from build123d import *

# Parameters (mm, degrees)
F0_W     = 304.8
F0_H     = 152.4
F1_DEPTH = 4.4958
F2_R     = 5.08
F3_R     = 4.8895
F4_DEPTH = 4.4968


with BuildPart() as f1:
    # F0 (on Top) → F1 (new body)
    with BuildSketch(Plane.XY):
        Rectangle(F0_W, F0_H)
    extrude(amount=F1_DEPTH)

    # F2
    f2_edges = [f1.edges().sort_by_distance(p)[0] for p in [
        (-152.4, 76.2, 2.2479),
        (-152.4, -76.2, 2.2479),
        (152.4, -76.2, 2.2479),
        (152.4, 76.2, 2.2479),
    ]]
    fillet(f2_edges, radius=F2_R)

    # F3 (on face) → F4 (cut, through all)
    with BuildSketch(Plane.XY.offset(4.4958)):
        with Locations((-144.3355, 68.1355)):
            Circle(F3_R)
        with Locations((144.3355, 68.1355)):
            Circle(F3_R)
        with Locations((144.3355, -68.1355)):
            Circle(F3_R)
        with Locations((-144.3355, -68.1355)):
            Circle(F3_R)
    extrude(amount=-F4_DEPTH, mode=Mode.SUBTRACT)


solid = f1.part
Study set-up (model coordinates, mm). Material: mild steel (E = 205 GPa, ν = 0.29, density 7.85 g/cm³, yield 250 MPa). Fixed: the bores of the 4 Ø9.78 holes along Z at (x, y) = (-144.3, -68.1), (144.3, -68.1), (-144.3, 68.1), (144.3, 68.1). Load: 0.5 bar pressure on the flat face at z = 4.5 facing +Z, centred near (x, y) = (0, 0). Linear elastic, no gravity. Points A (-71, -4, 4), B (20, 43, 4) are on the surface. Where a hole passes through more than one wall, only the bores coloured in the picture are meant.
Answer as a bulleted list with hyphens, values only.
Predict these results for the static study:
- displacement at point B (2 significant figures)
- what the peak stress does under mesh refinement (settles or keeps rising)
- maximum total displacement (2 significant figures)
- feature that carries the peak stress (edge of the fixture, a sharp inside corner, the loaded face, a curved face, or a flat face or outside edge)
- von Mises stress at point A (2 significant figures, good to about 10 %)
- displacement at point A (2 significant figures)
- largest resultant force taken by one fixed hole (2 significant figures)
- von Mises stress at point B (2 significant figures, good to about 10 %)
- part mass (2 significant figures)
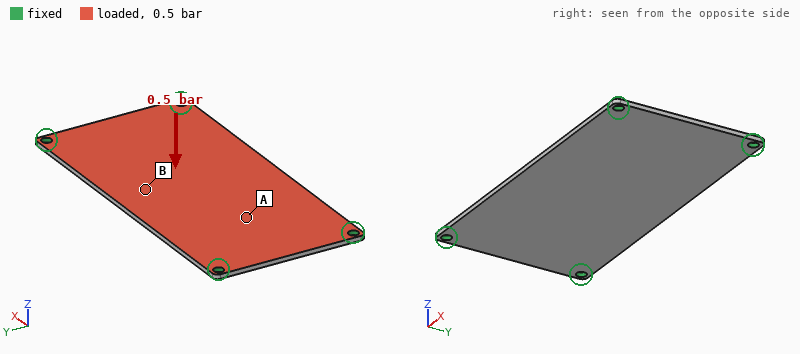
- 0.76 mm
- keeps rising
- 0.80 mm
- edge of the fixture
- 23 MPa
- 0.51 mm
- 580 N
- 55 MPa
- 1.6 kg
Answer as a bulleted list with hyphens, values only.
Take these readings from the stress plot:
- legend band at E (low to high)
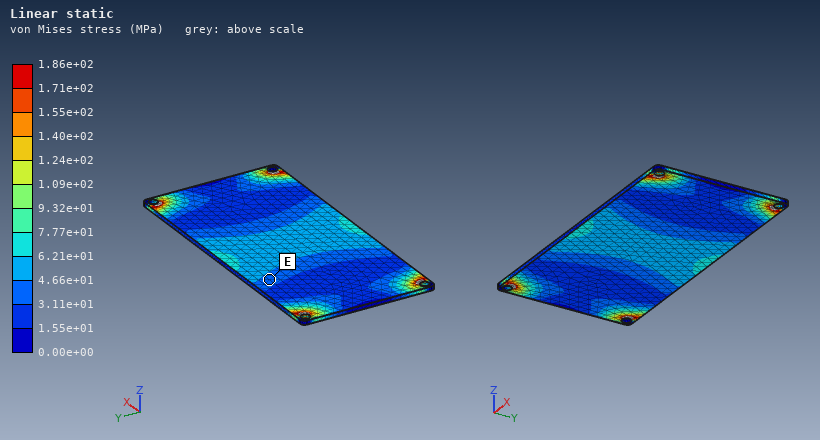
- 3.11e+01 to 4.66e+01 MPa
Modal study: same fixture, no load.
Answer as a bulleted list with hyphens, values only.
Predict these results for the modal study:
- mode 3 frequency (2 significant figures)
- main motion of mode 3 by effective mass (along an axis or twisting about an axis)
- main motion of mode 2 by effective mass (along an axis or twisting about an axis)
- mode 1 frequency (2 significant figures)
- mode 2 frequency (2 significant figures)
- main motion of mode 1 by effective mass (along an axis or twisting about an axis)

- 680 Hz
- twisting about Y
- twisting about X
- 240 Hz
- 460 Hz
- along Z
